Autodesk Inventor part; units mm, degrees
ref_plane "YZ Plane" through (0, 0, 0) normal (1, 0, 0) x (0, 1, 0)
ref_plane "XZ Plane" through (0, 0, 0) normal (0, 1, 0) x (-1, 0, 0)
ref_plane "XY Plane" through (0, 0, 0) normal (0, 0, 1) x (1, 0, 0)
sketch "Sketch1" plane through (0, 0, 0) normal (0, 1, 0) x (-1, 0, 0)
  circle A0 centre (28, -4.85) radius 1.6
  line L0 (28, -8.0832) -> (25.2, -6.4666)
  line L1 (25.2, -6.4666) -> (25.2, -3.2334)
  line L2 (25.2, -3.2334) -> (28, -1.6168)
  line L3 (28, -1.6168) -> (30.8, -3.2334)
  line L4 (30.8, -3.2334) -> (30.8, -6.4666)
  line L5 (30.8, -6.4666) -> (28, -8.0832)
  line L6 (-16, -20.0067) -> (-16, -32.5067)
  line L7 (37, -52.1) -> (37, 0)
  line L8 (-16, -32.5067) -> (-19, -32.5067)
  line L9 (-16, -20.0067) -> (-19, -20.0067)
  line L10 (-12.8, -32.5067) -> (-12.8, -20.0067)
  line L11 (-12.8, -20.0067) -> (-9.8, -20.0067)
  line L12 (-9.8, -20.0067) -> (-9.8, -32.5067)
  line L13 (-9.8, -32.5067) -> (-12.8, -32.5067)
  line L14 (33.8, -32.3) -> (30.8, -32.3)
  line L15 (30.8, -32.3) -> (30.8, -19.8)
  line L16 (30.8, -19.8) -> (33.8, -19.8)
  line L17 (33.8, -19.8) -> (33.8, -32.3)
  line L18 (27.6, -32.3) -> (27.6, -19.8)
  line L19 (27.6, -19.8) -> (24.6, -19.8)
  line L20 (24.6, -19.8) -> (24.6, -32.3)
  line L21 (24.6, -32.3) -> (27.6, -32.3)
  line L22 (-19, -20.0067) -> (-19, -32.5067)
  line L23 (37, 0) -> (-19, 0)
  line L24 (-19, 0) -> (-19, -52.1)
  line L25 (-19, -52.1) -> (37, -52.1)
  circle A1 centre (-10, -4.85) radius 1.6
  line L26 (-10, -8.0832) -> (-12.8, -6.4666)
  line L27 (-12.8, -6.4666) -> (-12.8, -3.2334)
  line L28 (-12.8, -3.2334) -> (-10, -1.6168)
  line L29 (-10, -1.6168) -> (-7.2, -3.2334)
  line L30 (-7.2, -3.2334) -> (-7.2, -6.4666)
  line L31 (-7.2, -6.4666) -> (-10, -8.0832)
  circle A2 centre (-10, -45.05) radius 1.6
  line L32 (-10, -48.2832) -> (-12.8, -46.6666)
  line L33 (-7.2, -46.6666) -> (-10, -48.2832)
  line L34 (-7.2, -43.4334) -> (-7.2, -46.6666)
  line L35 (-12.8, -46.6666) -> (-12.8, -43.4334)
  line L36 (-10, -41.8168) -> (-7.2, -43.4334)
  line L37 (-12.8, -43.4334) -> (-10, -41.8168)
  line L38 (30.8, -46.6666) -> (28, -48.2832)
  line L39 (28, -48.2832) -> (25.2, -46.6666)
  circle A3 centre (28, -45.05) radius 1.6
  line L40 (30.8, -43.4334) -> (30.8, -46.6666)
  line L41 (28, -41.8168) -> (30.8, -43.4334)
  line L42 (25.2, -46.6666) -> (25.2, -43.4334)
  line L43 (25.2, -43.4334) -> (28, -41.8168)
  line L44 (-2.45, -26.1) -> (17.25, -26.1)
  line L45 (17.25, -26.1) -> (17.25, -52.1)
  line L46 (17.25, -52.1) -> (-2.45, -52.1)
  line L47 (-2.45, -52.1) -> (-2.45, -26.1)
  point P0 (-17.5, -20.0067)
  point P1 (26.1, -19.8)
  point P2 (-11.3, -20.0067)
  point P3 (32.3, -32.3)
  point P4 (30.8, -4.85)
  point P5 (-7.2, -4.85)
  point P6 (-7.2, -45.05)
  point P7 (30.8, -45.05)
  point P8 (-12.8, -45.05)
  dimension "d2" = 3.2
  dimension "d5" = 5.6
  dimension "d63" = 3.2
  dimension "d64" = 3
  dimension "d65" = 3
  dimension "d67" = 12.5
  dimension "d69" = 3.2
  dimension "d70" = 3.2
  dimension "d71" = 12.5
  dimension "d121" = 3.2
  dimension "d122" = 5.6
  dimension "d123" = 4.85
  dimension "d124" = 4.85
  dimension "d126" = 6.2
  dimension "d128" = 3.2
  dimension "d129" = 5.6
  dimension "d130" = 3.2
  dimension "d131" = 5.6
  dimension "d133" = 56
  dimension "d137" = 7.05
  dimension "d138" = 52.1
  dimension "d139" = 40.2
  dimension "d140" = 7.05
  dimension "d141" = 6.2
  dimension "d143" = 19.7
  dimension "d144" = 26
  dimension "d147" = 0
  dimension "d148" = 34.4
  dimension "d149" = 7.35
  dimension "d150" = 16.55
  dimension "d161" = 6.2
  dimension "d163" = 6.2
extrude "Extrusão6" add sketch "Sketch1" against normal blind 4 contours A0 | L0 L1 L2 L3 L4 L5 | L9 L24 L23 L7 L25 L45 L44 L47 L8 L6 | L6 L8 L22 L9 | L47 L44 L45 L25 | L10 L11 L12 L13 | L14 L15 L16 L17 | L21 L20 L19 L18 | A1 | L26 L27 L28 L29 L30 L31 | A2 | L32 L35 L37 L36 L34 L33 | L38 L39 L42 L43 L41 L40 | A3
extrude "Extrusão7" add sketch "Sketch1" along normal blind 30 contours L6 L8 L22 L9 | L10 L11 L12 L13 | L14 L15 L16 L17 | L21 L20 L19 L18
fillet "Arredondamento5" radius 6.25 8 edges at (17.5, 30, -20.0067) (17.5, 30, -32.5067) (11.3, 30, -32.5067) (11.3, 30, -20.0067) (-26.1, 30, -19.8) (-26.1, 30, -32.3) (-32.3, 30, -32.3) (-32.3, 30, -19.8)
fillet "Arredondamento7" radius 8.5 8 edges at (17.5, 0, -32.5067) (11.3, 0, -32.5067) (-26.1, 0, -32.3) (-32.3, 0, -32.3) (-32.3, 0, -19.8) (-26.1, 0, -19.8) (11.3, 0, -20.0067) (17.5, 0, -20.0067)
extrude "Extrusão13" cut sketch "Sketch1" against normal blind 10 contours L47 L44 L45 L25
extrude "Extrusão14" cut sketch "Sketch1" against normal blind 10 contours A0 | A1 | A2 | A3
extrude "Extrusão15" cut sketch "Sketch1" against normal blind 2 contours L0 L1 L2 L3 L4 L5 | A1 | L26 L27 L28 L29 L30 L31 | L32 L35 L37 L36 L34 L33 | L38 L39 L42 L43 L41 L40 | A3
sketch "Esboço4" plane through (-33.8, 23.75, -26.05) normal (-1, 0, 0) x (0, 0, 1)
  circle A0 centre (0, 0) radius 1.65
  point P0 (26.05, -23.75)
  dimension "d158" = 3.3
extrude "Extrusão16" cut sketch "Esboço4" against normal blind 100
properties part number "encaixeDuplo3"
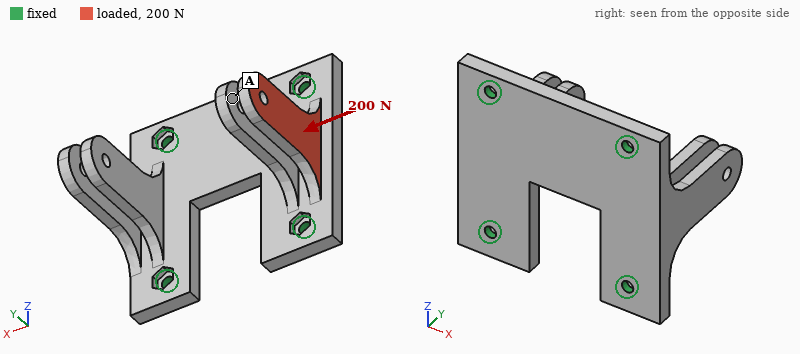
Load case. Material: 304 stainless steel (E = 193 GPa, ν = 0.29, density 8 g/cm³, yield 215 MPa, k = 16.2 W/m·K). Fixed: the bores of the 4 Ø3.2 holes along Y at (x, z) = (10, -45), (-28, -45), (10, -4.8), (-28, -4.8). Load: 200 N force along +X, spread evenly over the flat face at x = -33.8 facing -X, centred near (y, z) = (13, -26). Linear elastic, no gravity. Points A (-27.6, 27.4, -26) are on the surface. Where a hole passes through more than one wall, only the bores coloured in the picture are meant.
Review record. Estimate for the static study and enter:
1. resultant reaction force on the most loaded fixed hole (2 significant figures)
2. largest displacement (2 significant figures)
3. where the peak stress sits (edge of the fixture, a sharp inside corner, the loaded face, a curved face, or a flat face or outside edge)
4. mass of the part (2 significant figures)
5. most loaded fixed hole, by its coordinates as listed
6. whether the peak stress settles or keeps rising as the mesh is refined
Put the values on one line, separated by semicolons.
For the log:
190 N; 0.13 mm; edge of the fixture; 110 g; (10, -4.8); keeps rising
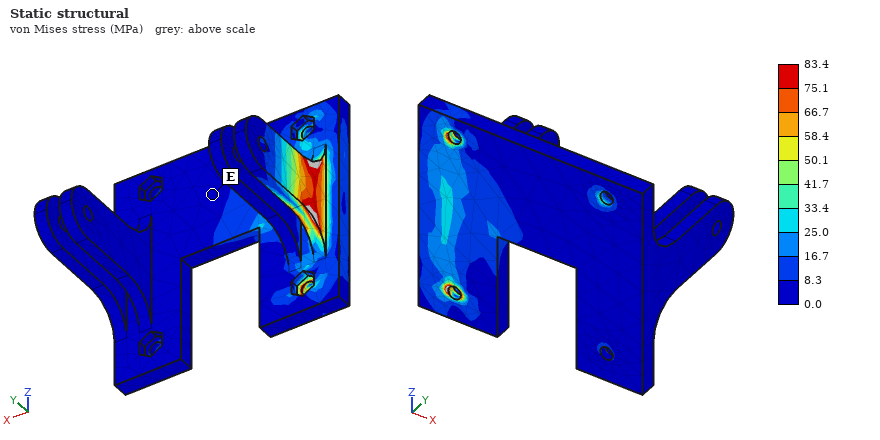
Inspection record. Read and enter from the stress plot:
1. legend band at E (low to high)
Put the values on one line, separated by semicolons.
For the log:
0.0 to 8.3 MPa
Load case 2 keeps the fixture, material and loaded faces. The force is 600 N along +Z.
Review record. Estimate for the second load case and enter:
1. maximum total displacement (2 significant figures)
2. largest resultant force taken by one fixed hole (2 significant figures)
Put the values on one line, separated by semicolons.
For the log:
30 µm; 430 N
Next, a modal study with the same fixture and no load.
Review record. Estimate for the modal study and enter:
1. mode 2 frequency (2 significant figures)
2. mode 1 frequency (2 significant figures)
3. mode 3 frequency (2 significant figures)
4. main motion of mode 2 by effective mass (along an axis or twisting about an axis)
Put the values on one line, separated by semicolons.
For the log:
2500 Hz; 2400 Hz; 2900 Hz; along X
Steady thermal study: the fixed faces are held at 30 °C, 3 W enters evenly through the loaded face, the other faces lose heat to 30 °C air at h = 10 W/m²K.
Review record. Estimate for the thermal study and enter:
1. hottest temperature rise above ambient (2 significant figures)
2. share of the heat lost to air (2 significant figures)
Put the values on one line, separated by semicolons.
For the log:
73 K; 25 %
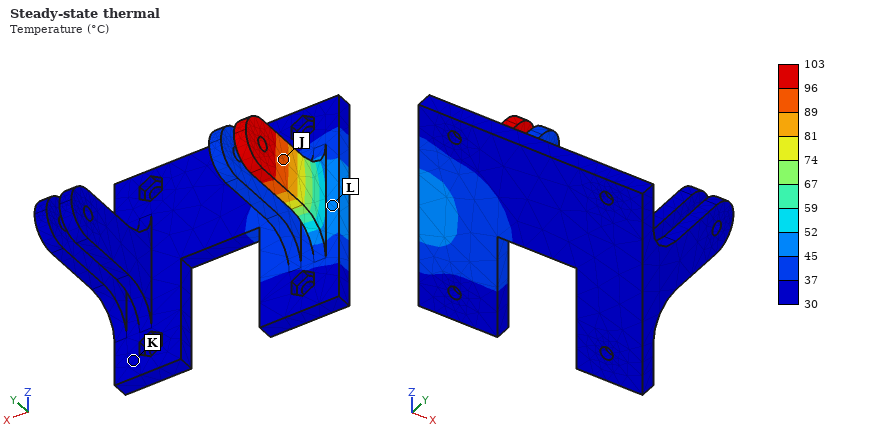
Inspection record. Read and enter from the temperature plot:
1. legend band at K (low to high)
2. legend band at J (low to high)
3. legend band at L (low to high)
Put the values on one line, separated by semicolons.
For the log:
30 to 37 °C; 89 to 96 °C; 45 to 52 °C
